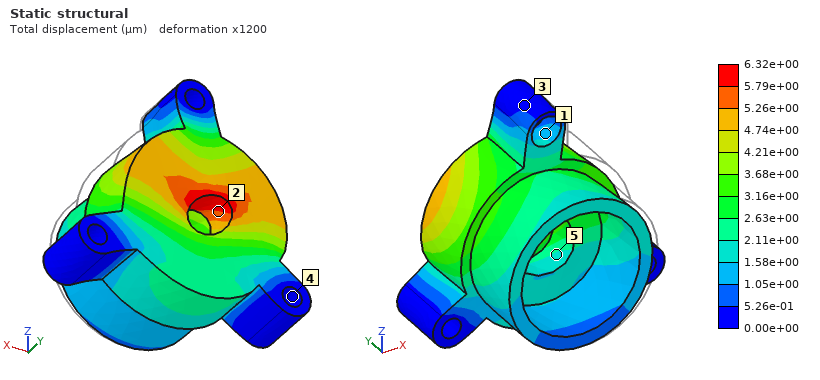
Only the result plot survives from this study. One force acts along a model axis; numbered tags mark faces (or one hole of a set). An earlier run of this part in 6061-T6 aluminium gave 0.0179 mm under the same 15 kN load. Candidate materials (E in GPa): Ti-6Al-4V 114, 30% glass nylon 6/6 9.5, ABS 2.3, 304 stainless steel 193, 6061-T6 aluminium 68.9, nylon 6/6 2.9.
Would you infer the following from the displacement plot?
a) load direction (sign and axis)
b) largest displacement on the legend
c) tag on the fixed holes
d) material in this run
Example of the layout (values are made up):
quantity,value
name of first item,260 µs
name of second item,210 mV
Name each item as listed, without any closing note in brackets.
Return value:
quantity,value
load direction,-X
largest displacement on the legend,6.32e+00 µm
tag on the fixed holes,4
material in this run,304 stainless steel
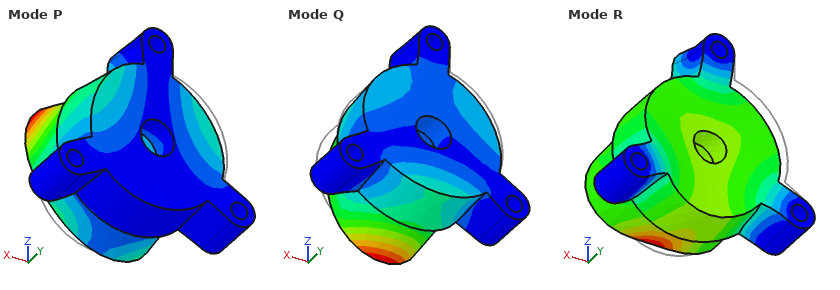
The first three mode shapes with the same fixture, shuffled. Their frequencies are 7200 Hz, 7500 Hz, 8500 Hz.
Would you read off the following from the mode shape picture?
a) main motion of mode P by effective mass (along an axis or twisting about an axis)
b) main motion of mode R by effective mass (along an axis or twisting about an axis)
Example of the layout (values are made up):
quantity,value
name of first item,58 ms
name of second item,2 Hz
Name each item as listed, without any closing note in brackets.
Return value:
quantity,value
main motion of mode P by effective mass,along X
main motion of mode R by effective mass,along Y
